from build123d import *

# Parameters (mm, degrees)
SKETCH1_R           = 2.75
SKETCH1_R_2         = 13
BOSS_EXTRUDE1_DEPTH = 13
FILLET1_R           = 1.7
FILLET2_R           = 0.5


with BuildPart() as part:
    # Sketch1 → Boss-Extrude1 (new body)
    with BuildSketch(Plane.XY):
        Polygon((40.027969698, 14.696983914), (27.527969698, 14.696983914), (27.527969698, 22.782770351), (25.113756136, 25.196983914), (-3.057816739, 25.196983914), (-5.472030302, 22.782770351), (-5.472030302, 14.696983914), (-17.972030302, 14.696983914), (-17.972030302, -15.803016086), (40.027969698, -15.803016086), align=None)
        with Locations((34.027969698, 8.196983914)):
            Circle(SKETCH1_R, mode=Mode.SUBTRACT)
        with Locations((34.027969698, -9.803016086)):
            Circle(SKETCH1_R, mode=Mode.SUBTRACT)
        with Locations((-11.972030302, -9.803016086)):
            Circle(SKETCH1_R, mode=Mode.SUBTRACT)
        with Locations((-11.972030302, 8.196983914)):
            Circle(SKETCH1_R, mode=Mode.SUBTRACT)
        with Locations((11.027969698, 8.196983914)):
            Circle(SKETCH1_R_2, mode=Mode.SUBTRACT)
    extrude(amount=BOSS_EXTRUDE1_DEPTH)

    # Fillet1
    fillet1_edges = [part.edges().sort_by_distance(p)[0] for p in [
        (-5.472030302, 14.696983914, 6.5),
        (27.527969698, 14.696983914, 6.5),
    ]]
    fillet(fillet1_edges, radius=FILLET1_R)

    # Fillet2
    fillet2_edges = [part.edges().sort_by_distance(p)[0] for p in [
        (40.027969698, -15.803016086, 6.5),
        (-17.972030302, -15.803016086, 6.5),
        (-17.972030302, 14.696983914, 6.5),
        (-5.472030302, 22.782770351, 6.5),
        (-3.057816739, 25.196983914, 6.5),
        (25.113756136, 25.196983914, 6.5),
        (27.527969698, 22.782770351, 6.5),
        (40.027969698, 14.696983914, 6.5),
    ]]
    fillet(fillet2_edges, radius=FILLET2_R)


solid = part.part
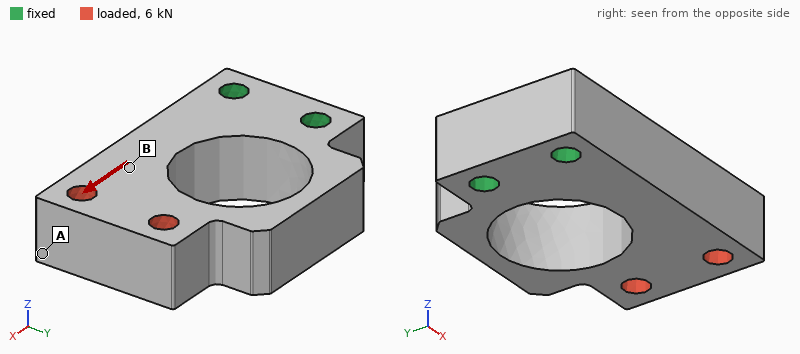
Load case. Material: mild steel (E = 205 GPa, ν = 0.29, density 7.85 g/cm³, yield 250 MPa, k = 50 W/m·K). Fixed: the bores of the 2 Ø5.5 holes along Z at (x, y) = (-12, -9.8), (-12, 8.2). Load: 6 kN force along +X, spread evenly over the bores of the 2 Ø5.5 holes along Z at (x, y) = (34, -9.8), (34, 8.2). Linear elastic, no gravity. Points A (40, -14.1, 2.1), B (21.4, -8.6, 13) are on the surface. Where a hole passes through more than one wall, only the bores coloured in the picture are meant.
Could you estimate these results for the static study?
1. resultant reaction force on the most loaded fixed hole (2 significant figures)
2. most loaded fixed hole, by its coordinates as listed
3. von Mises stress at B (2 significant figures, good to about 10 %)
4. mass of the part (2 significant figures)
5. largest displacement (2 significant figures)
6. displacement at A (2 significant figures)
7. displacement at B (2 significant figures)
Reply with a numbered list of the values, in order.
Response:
1. 3.3 kN
2. (-12, -9.8)
3. 34 MPa
4. 150 g
5. 38 µm
6. 28 µm
7. 11 µm
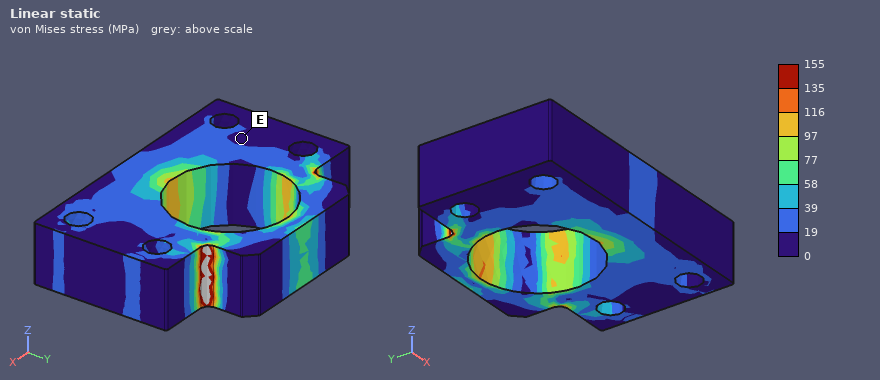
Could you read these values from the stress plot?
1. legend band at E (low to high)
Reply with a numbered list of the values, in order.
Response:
1. 0 to 19 MPa
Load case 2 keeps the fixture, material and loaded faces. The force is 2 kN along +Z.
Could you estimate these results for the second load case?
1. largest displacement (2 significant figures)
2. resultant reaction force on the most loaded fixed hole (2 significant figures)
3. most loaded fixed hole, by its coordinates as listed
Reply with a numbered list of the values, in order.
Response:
1. 0.12 mm
2. 1.1 kN
3. (-12, -9.8)
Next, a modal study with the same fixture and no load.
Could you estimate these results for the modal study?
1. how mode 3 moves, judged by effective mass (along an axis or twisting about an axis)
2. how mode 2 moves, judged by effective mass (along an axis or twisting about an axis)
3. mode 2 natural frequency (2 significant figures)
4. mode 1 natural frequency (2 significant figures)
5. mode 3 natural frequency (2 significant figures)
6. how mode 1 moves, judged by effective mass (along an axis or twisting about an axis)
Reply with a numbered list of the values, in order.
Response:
1. twisting about X
2. along Y
3. 4400 Hz
4. 3200 Hz
5. 7700 Hz
6. along Z
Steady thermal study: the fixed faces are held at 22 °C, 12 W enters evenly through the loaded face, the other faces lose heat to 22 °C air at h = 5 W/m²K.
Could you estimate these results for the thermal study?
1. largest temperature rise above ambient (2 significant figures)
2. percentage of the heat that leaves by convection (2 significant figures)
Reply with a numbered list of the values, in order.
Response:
1. 43 K
2. 5.5 %
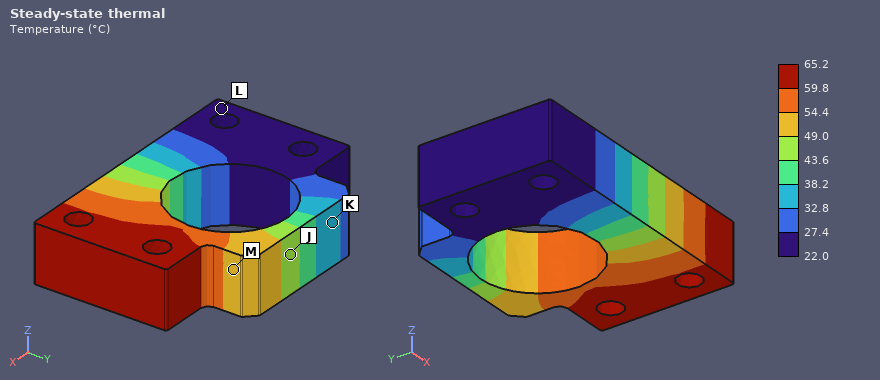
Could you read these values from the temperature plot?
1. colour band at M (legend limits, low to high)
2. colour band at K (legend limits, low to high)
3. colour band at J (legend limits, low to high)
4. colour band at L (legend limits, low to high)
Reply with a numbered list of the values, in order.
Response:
1. 49.0 to 54.4 °C
2. 32.8 to 38.2 °C
3. 43.6 to 49.0 °C
4. 22.0 to 27.4 °C
